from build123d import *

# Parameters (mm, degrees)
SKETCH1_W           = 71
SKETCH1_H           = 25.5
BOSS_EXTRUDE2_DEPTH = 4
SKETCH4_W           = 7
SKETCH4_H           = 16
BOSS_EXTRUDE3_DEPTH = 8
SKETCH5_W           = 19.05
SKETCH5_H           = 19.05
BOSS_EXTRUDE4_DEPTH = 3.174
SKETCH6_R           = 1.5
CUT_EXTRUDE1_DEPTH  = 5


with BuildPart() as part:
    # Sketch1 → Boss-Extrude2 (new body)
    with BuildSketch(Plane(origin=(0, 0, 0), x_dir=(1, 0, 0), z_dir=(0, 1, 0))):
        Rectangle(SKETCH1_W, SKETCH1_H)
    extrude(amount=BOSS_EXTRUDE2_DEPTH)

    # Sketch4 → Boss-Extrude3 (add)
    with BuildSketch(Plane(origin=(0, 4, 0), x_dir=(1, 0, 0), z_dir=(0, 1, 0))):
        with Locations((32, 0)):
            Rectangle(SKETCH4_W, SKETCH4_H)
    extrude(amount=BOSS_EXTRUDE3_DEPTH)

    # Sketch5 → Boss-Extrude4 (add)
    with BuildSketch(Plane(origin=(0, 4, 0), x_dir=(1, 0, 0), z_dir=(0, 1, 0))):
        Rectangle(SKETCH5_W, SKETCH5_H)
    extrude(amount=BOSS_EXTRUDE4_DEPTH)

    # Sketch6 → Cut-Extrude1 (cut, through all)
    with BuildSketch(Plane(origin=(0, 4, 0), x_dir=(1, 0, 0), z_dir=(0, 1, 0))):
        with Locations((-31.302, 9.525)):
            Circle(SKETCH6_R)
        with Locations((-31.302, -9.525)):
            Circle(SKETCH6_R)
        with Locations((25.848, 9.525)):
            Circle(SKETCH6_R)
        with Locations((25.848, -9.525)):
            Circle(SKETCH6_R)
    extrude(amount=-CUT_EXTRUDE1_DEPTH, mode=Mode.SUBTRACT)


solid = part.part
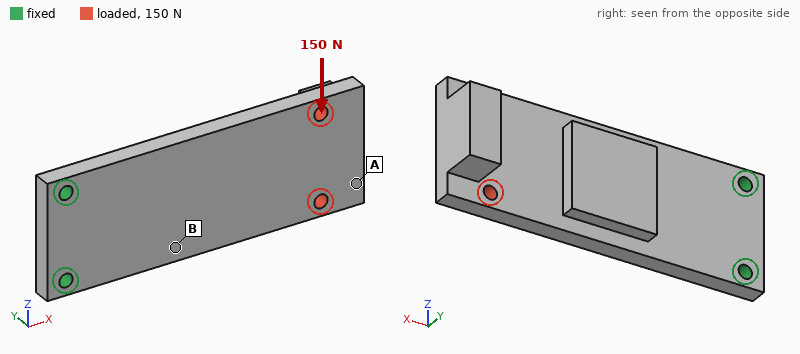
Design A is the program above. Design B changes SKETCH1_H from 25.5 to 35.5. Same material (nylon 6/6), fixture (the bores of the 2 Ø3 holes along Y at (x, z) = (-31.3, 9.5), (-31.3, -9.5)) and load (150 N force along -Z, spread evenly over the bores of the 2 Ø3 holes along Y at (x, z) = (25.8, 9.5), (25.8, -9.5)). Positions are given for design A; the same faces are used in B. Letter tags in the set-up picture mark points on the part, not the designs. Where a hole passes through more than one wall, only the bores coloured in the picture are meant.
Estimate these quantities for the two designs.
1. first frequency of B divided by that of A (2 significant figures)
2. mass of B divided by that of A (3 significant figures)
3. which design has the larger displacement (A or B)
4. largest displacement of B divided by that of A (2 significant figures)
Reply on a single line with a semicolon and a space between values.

1.0; 1.31; A; 0.58
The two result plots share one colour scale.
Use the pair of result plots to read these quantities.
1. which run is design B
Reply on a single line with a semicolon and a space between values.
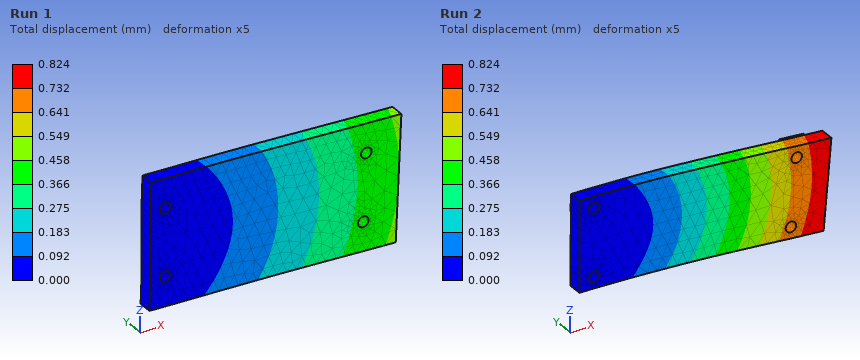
Run 1
